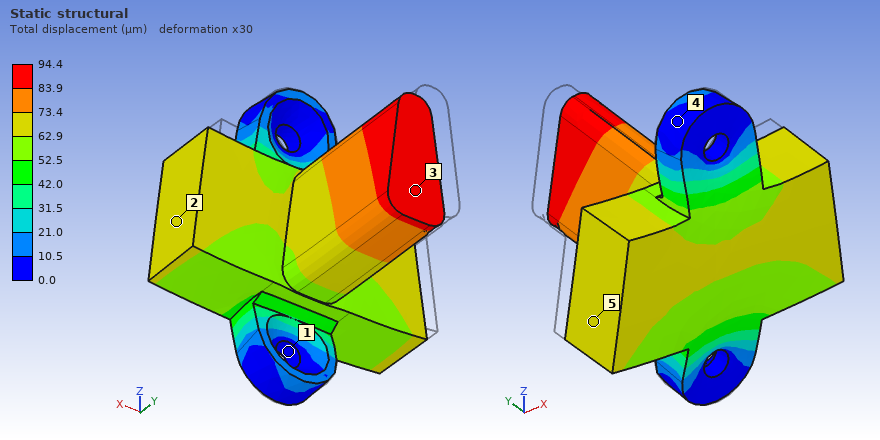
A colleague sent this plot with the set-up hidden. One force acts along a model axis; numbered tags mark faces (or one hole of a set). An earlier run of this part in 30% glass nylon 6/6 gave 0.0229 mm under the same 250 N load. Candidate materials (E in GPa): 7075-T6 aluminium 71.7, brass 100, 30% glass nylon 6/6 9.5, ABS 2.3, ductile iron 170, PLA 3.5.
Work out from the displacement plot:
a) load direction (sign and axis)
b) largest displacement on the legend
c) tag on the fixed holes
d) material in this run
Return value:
-Y
94.4 µm
1
ABS
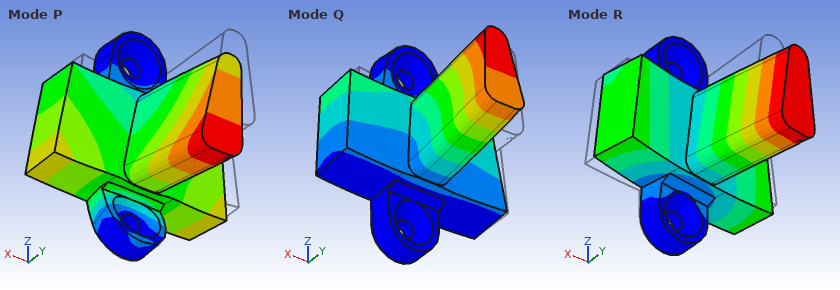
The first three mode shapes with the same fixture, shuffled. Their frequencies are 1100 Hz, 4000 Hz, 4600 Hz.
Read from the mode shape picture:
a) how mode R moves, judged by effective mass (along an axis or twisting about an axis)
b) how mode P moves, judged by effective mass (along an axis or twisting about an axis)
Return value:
along X
along Y
